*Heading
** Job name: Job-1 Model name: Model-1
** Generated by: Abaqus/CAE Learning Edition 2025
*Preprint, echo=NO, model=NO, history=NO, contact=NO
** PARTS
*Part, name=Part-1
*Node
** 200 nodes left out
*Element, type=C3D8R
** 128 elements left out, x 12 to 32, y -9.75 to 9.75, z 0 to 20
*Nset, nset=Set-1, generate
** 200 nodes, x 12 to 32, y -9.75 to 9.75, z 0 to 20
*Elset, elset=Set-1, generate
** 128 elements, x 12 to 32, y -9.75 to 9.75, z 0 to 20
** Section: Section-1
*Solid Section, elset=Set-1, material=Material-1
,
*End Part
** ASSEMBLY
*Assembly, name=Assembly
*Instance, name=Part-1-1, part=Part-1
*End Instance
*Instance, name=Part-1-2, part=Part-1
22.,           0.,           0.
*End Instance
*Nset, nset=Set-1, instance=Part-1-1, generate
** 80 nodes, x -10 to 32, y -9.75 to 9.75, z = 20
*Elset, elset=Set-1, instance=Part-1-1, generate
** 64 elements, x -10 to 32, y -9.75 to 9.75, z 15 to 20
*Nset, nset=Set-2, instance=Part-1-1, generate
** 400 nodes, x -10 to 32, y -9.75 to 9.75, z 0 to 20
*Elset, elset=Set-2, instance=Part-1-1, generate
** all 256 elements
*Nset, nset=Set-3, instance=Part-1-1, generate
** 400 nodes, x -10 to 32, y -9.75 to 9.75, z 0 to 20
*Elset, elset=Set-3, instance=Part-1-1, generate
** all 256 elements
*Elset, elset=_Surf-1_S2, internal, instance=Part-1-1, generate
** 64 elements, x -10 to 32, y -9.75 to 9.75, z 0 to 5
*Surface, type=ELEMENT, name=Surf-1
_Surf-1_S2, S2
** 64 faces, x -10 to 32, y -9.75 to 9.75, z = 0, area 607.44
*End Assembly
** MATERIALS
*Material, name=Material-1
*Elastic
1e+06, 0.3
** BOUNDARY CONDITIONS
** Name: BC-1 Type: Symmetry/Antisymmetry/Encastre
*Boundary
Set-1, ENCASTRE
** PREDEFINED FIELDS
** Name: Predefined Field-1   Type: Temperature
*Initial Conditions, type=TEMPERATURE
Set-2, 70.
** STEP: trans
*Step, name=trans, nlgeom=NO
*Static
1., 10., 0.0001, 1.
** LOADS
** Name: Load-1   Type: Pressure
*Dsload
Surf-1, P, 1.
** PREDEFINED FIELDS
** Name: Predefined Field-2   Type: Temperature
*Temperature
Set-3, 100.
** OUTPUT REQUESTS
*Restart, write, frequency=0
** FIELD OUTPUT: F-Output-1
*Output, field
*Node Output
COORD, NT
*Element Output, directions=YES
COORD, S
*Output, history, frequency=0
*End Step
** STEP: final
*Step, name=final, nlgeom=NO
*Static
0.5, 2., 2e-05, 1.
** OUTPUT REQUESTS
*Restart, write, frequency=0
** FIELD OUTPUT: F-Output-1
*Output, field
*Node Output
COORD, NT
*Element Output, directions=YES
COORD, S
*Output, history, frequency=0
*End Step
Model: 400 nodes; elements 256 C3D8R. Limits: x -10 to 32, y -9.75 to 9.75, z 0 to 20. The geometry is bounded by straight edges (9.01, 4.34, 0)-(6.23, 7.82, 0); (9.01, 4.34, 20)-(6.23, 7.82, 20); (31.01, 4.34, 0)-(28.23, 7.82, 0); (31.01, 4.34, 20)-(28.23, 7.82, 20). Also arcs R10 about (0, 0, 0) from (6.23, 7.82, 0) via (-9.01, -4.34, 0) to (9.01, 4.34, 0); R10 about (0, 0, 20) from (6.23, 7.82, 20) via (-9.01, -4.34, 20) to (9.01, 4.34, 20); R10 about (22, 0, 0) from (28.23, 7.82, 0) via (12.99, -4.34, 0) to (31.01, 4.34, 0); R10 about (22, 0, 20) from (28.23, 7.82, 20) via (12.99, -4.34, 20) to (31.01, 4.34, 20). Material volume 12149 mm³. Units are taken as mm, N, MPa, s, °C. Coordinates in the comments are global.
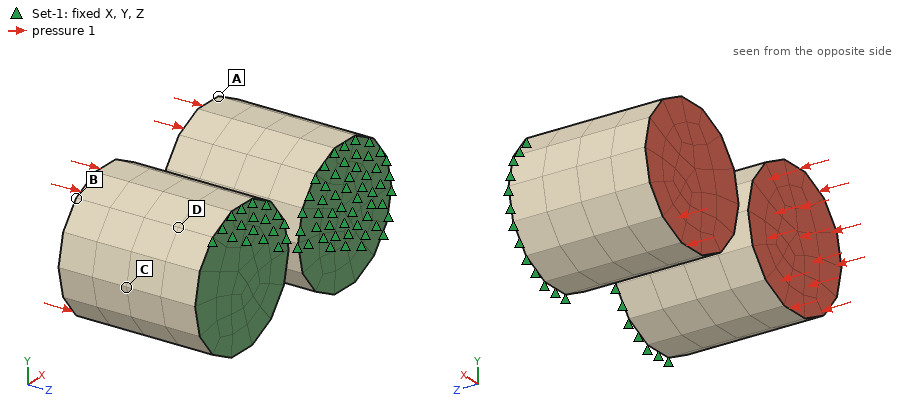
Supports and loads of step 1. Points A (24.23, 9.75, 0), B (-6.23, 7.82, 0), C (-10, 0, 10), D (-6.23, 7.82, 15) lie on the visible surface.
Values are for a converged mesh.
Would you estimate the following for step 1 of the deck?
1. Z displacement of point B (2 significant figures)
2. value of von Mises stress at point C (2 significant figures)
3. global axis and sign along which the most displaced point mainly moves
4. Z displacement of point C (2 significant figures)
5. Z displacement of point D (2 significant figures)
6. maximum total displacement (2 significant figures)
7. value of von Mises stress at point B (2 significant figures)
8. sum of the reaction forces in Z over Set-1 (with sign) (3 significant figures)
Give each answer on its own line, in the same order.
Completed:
1.9e-05 mm
0.97 MPa
+Z
9.6e-06 mm
4.9e-06 mm
2.0e-05 mm
1.0 MPa
-607 N
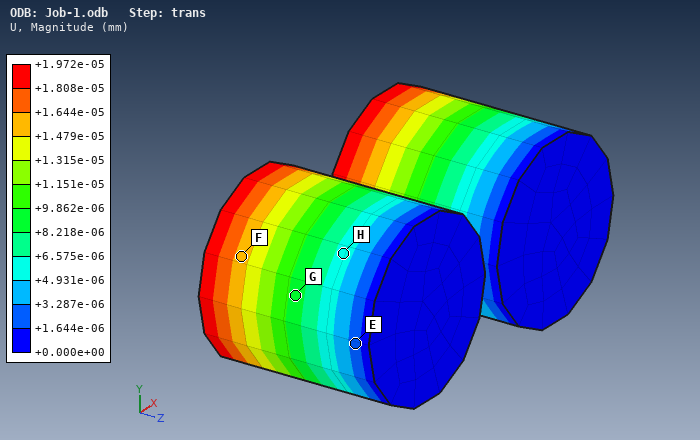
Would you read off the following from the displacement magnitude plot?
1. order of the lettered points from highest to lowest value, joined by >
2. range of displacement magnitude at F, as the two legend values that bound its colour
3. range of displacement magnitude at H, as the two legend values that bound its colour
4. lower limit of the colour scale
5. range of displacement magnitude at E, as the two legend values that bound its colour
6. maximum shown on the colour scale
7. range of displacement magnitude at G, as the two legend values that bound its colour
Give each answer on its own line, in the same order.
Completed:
F > G > H > E
+1.479e-05 to +1.644e-05 mm
+4.931e-06 to +6.575e-06 mm
+0.000e+00 mm
+1.644e-06 to +3.287e-06 mm
+1.972e-05 mm
+8.218e-06 to +9.862e-06 mm
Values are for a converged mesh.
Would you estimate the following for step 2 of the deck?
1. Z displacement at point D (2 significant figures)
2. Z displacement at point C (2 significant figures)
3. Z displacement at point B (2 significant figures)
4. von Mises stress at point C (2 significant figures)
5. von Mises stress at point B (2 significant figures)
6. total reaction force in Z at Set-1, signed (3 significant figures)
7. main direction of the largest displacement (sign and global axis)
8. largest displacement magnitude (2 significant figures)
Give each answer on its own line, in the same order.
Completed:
4.9e-06 mm
9.6e-06 mm
1.9e-05 mm
0.97 MPa
1.0 MPa
-607 N
+Z
2.0e-05 mm
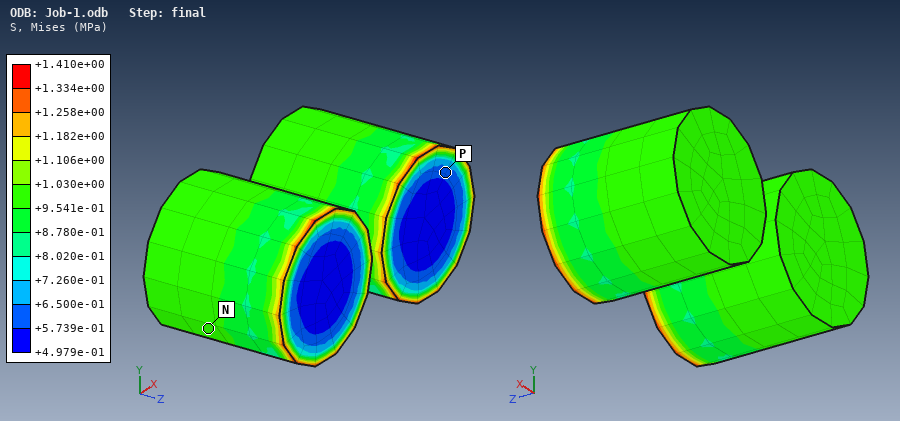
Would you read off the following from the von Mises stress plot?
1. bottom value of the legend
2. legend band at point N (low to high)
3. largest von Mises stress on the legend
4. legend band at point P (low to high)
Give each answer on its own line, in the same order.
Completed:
+4.979e-01 MPa
+9.541e-01 to +1.030e+00 MPa
+1.410e+00 MPa
+5.739e-01 to +6.500e-01 MPa
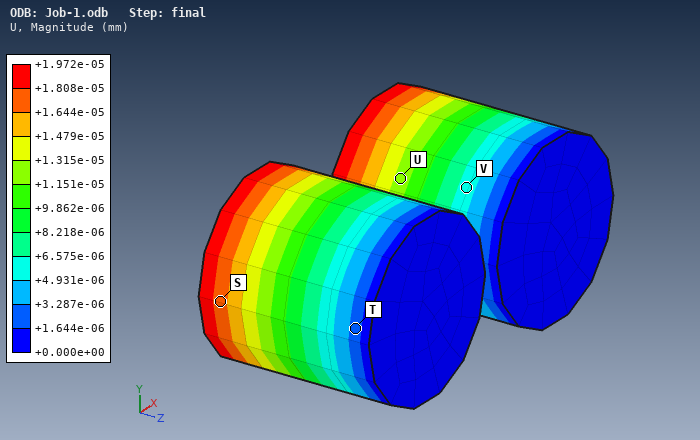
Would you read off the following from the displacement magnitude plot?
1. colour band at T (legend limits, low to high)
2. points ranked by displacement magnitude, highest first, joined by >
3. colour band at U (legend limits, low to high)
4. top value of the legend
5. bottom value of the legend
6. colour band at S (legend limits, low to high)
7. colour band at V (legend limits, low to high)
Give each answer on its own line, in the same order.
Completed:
+1.644e-06 to +3.287e-06 mm
S > U > V > T
+1.151e-05 to +1.315e-05 mm
+1.972e-05 mm
+0.000e+00 mm
+1.644e-05 to +1.808e-05 mm
+4.931e-06 to +6.575e-06 mm
